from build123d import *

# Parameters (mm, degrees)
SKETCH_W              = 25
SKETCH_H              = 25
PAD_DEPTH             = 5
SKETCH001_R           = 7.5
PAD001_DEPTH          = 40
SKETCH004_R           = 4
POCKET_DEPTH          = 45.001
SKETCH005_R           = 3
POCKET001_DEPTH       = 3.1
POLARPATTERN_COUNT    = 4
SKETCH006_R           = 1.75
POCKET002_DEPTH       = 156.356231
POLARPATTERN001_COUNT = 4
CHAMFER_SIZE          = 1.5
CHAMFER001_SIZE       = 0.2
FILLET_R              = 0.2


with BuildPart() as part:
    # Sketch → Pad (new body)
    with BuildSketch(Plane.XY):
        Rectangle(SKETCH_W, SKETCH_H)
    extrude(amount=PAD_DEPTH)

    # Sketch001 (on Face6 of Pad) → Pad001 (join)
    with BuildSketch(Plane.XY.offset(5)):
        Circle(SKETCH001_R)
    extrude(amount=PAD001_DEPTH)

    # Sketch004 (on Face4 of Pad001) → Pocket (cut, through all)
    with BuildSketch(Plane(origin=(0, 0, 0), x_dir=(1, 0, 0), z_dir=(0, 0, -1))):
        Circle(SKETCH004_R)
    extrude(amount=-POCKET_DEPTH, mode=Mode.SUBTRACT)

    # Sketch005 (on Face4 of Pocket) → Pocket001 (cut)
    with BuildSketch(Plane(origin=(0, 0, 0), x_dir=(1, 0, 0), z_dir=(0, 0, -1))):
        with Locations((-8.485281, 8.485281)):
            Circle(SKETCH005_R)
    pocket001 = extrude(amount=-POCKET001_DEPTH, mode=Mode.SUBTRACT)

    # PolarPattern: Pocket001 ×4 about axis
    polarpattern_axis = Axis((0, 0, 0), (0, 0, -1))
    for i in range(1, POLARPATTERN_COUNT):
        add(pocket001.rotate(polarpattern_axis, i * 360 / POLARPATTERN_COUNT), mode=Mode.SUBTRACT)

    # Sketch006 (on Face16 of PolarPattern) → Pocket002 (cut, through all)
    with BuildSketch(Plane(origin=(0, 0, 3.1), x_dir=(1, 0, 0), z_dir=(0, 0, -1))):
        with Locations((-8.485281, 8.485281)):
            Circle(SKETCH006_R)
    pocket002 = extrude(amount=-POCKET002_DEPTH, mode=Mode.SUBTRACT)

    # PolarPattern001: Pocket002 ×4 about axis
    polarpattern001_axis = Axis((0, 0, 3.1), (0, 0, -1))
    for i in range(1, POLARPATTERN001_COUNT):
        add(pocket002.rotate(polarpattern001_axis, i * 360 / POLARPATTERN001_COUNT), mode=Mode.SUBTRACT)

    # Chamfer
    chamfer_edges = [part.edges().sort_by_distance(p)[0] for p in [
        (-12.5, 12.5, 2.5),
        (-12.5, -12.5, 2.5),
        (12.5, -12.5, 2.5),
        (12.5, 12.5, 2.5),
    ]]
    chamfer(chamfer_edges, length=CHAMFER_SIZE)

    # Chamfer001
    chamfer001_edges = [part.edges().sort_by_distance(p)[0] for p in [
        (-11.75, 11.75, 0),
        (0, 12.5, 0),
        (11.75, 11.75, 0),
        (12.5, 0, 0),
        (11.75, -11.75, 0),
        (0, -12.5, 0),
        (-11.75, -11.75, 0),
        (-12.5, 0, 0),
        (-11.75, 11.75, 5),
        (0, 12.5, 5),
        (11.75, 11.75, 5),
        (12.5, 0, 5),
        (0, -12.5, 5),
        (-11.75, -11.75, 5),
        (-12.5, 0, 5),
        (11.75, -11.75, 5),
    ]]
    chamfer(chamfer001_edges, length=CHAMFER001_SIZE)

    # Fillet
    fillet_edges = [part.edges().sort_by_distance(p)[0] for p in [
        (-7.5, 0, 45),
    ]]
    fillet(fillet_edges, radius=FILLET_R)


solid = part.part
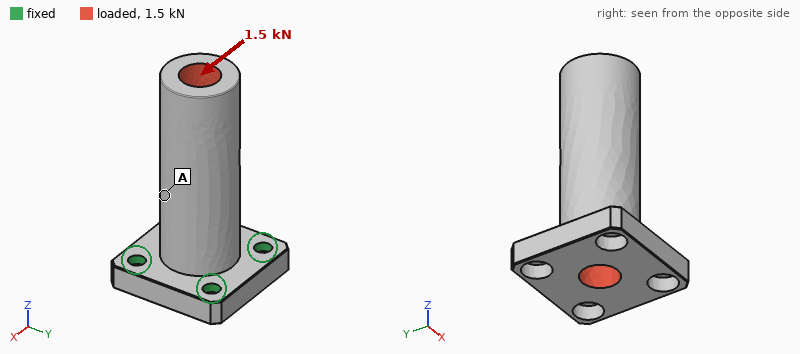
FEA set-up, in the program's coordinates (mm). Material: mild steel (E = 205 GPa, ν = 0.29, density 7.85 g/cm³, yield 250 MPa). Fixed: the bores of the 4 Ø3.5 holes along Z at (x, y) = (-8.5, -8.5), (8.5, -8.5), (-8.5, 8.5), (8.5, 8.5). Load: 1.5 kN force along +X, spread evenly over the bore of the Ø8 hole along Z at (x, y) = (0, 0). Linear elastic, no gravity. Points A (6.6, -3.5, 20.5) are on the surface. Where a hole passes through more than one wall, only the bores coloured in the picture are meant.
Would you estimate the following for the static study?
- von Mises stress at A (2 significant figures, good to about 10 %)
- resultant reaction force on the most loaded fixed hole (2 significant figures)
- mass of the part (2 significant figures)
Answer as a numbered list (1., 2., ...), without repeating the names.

1. 30 MPa
2. 950 N
3. 59 g
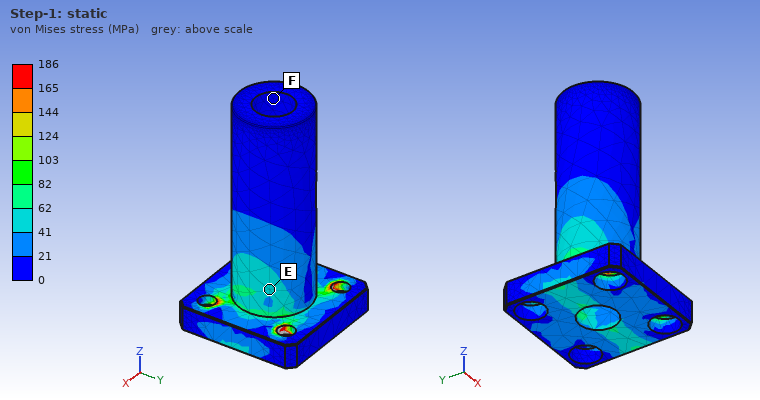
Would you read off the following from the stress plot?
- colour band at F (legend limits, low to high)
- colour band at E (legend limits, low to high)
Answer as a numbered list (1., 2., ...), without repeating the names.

1. 0 to 21 MPa
2. 41 to 62 MPa
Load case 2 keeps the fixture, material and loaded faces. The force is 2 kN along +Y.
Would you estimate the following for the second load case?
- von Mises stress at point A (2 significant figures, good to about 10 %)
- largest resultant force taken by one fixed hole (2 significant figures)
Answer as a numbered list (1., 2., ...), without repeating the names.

1. 29 MPa
2. 1.3 kN
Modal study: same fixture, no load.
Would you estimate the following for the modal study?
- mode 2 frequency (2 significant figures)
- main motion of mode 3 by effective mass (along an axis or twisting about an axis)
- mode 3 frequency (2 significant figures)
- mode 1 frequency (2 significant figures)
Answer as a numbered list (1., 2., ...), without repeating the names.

1. 4900 Hz
2. along Z
3. 19 kHz
4. 4800 Hz
